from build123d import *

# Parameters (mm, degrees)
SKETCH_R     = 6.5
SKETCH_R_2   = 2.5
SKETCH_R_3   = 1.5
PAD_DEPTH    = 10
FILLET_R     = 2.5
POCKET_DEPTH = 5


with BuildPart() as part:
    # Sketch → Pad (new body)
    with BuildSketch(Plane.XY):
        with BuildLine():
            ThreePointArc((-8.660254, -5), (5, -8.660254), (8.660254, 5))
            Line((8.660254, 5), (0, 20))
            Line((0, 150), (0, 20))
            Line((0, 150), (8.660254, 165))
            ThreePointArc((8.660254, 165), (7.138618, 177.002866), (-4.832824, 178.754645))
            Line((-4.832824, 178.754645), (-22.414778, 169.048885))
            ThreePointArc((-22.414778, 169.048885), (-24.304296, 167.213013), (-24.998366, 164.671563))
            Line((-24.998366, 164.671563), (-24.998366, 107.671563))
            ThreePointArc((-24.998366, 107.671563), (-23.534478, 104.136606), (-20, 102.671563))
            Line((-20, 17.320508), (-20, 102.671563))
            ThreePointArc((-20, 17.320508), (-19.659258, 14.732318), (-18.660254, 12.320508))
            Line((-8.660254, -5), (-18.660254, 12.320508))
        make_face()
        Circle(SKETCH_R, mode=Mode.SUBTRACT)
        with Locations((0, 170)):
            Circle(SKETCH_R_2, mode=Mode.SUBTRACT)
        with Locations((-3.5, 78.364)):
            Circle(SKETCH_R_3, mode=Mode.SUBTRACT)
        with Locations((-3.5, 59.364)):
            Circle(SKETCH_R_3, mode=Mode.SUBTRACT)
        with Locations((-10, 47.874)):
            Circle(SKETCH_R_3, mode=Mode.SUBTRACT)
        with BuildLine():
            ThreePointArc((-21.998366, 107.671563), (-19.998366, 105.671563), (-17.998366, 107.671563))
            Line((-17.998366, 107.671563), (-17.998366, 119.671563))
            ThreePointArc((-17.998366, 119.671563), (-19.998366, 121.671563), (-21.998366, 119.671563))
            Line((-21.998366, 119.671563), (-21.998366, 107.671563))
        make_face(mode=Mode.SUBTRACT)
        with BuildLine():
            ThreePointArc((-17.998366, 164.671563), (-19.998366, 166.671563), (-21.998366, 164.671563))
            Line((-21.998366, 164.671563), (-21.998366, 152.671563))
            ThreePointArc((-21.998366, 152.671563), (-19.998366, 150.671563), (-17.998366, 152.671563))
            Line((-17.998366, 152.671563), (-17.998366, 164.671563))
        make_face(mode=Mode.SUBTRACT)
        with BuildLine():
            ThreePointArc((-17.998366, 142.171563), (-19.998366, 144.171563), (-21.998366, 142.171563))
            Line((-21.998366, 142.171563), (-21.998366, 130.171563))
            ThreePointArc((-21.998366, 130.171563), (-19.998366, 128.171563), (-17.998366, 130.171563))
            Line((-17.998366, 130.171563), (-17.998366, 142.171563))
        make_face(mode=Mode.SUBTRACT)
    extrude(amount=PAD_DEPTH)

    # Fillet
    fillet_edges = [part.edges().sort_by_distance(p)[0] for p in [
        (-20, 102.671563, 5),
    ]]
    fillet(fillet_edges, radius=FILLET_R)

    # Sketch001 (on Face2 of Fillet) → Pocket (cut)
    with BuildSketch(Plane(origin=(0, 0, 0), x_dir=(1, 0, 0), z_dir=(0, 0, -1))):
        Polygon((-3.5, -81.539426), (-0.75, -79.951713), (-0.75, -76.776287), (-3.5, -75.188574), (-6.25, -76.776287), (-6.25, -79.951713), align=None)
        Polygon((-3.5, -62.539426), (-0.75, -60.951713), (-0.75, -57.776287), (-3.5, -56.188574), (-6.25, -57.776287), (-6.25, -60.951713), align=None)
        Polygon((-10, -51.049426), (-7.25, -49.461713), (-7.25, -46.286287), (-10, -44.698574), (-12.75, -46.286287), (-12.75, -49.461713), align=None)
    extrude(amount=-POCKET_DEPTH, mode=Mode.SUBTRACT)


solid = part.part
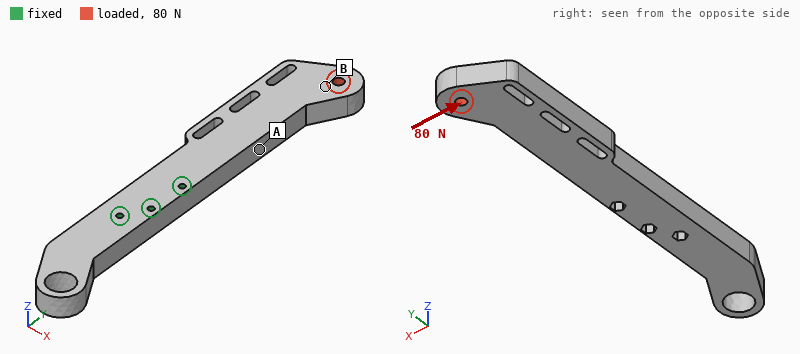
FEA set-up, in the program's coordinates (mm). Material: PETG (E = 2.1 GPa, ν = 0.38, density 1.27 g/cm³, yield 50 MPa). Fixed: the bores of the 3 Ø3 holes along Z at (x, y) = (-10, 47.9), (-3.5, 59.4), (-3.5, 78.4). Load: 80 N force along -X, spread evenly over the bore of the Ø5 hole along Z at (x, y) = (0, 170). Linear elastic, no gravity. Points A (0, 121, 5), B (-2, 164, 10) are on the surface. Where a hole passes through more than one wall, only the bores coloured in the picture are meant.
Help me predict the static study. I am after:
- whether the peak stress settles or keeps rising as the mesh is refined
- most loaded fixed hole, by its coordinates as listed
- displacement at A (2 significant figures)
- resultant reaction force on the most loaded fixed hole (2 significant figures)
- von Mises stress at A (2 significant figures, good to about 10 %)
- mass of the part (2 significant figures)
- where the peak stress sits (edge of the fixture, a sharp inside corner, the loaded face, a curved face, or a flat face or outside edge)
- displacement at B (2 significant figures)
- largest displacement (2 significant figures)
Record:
keeps rising
(-3.5, 78.4)
0.75 mm
420 N
4.8 MPa
49 g
edge of the fixture
1.9 mm
2.3 mm
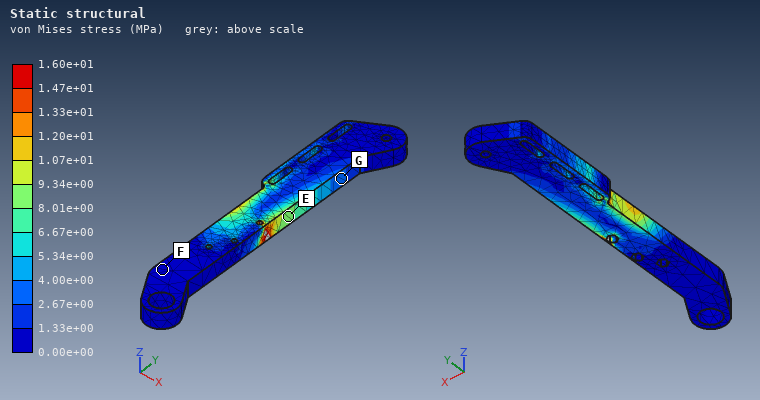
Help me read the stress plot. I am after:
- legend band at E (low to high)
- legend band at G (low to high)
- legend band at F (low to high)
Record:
8.01e+00 to 9.34e+00 MPa
2.67e+00 to 4.00e+00 MPa
0.00e+00 to 1.33e+00 MPa
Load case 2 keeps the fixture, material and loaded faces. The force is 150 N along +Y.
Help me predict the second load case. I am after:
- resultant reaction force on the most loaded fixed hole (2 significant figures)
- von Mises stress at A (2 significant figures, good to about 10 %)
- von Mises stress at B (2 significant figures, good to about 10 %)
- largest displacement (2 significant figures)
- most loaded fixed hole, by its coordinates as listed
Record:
140 N
2.7 MPa
1.3 MPa
0.59 mm
(-3.5, 78.4)
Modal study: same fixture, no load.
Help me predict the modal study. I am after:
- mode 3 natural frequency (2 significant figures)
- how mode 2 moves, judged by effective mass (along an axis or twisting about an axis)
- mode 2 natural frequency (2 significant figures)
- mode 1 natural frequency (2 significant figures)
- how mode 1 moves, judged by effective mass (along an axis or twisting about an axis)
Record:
580 Hz
along X
310 Hz
160 Hz
along Z
